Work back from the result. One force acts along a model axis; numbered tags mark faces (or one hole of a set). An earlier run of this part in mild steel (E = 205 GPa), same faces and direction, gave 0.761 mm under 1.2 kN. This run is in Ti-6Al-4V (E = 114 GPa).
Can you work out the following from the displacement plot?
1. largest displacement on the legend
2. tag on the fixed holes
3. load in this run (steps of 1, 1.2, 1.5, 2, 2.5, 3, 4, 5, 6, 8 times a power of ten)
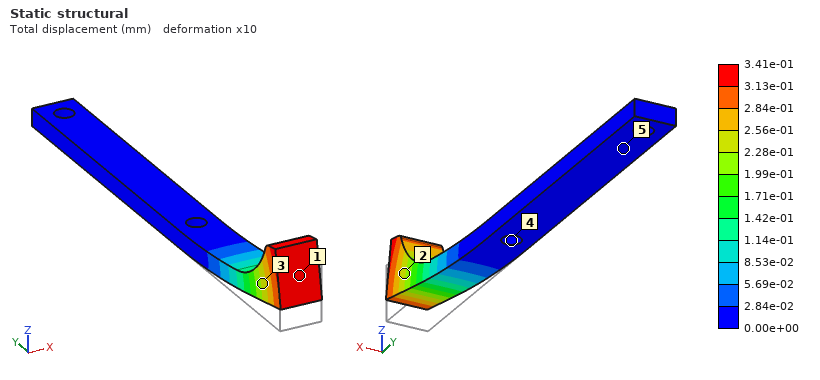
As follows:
3.41e-01 mm
4
300 N
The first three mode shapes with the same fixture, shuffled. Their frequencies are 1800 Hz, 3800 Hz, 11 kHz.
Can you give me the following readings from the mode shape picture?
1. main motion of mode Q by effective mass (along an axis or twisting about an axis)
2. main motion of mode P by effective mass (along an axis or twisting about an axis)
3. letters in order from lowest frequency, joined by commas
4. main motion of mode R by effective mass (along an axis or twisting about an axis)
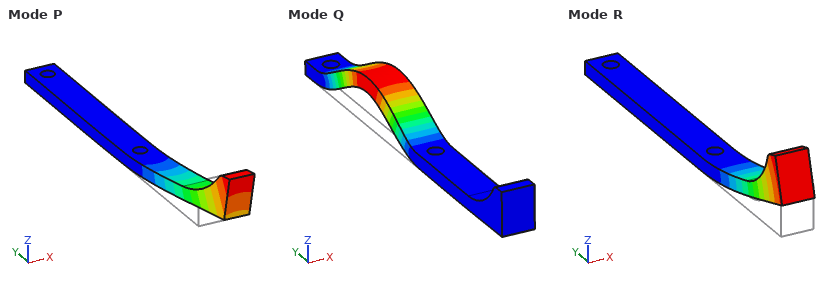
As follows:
along Z
along X
R, P, Q
along Z
